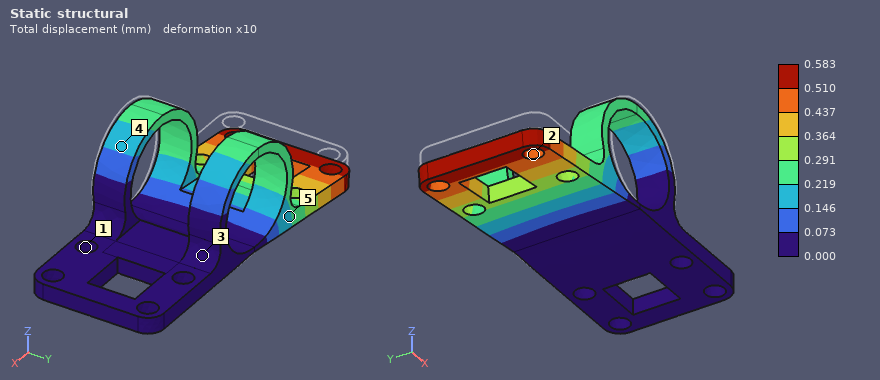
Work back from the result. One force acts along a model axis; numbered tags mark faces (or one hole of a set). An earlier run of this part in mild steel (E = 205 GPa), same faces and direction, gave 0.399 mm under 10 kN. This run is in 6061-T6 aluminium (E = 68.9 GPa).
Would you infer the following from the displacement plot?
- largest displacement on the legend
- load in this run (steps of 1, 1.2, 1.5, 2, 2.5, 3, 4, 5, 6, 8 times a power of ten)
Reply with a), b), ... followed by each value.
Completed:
a) 0.583 mm
b) 5 kN
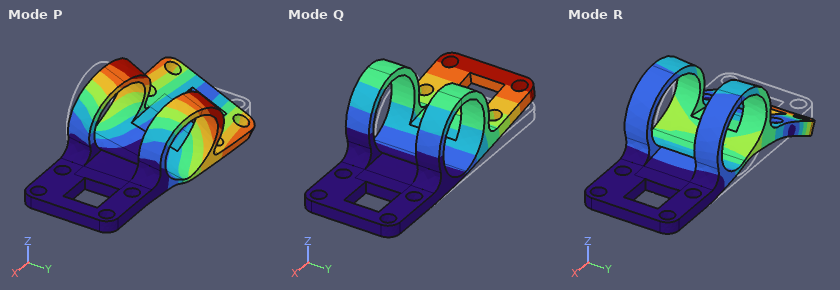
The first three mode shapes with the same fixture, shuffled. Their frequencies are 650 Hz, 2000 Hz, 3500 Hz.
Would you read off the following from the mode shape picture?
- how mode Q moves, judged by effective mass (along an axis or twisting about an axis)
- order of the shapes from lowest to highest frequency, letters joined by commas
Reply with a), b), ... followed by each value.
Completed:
a) along Z
b) Q, P, R
